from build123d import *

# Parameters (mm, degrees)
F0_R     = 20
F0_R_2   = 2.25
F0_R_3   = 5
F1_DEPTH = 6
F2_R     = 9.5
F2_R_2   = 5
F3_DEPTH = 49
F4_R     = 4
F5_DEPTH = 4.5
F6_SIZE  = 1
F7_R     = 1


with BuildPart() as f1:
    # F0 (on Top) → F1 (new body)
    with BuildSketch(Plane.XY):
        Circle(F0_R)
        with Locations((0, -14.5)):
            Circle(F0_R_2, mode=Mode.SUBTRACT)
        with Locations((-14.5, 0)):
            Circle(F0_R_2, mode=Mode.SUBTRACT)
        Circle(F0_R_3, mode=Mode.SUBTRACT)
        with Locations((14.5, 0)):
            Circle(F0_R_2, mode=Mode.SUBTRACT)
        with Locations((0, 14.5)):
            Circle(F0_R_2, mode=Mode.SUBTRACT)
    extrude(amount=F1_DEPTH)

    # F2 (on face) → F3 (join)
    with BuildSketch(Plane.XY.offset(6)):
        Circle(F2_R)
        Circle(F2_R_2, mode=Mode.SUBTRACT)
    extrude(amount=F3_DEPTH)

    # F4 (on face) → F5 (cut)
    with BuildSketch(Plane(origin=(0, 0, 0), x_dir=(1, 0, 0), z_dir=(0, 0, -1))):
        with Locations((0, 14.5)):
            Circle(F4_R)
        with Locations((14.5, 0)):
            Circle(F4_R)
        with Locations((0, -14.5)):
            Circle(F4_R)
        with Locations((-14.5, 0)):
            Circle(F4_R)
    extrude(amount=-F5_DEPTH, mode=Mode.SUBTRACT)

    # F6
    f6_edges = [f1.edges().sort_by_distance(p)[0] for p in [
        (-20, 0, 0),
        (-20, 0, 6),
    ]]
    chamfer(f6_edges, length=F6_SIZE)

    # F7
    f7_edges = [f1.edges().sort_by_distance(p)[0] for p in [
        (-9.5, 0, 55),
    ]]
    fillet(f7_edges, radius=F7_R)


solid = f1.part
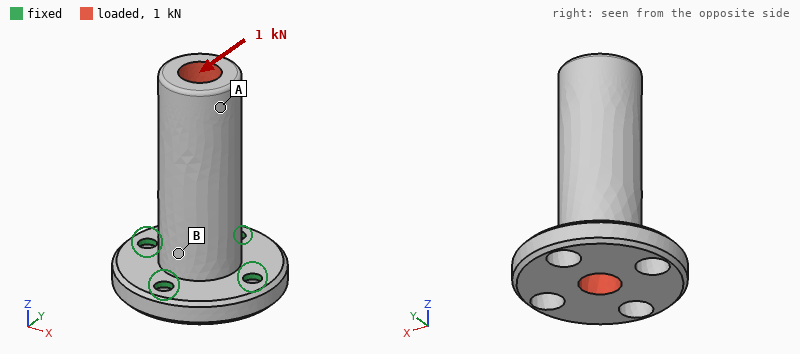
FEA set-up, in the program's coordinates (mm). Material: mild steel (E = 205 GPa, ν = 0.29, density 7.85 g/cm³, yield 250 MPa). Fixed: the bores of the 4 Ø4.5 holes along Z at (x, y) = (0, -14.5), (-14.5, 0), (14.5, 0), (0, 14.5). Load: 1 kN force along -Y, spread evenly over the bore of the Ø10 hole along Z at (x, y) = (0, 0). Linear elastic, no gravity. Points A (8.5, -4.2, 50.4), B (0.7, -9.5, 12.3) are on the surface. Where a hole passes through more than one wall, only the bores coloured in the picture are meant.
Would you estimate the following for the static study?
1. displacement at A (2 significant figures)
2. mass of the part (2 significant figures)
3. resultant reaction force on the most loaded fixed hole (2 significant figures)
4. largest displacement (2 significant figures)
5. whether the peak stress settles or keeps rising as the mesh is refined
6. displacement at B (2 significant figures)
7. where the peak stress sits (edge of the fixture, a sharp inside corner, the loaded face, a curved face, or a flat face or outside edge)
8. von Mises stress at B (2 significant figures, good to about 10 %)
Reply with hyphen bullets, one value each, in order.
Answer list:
- 26 µm
- 130 g
- 790 N
- 29 µm
- keeps rising
- 5.2 µm
- edge of the fixture
- 26 MPa
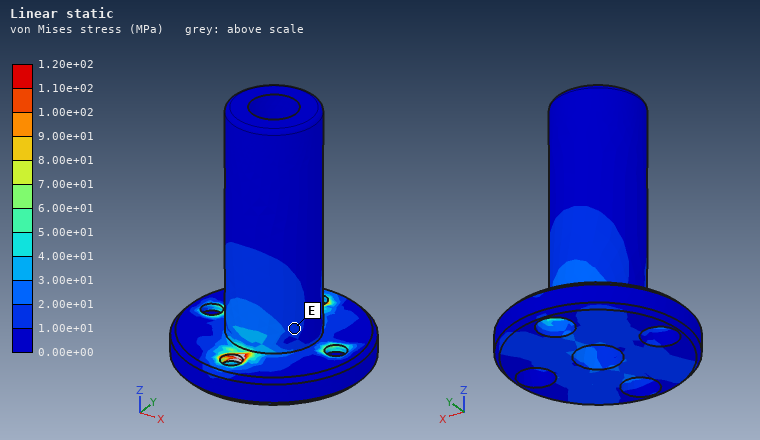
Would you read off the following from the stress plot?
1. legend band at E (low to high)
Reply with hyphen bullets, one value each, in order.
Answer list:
- 1.00e+01 to 2.00e+01 MPa
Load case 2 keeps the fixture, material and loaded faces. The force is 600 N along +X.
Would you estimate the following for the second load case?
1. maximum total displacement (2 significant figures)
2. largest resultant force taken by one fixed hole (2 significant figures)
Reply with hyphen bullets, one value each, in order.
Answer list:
- 17 µm
- 480 N
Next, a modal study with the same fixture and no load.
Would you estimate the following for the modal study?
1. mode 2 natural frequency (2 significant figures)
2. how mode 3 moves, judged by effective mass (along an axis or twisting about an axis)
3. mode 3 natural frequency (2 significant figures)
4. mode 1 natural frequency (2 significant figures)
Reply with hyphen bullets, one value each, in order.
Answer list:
- 3800 Hz
- along Z
- 14 kHz
- 3800 Hz
